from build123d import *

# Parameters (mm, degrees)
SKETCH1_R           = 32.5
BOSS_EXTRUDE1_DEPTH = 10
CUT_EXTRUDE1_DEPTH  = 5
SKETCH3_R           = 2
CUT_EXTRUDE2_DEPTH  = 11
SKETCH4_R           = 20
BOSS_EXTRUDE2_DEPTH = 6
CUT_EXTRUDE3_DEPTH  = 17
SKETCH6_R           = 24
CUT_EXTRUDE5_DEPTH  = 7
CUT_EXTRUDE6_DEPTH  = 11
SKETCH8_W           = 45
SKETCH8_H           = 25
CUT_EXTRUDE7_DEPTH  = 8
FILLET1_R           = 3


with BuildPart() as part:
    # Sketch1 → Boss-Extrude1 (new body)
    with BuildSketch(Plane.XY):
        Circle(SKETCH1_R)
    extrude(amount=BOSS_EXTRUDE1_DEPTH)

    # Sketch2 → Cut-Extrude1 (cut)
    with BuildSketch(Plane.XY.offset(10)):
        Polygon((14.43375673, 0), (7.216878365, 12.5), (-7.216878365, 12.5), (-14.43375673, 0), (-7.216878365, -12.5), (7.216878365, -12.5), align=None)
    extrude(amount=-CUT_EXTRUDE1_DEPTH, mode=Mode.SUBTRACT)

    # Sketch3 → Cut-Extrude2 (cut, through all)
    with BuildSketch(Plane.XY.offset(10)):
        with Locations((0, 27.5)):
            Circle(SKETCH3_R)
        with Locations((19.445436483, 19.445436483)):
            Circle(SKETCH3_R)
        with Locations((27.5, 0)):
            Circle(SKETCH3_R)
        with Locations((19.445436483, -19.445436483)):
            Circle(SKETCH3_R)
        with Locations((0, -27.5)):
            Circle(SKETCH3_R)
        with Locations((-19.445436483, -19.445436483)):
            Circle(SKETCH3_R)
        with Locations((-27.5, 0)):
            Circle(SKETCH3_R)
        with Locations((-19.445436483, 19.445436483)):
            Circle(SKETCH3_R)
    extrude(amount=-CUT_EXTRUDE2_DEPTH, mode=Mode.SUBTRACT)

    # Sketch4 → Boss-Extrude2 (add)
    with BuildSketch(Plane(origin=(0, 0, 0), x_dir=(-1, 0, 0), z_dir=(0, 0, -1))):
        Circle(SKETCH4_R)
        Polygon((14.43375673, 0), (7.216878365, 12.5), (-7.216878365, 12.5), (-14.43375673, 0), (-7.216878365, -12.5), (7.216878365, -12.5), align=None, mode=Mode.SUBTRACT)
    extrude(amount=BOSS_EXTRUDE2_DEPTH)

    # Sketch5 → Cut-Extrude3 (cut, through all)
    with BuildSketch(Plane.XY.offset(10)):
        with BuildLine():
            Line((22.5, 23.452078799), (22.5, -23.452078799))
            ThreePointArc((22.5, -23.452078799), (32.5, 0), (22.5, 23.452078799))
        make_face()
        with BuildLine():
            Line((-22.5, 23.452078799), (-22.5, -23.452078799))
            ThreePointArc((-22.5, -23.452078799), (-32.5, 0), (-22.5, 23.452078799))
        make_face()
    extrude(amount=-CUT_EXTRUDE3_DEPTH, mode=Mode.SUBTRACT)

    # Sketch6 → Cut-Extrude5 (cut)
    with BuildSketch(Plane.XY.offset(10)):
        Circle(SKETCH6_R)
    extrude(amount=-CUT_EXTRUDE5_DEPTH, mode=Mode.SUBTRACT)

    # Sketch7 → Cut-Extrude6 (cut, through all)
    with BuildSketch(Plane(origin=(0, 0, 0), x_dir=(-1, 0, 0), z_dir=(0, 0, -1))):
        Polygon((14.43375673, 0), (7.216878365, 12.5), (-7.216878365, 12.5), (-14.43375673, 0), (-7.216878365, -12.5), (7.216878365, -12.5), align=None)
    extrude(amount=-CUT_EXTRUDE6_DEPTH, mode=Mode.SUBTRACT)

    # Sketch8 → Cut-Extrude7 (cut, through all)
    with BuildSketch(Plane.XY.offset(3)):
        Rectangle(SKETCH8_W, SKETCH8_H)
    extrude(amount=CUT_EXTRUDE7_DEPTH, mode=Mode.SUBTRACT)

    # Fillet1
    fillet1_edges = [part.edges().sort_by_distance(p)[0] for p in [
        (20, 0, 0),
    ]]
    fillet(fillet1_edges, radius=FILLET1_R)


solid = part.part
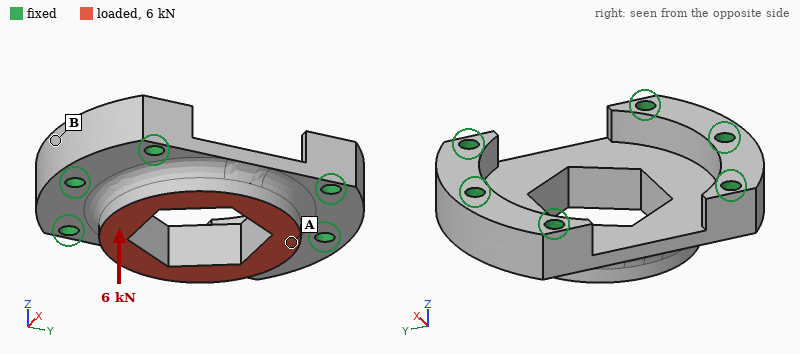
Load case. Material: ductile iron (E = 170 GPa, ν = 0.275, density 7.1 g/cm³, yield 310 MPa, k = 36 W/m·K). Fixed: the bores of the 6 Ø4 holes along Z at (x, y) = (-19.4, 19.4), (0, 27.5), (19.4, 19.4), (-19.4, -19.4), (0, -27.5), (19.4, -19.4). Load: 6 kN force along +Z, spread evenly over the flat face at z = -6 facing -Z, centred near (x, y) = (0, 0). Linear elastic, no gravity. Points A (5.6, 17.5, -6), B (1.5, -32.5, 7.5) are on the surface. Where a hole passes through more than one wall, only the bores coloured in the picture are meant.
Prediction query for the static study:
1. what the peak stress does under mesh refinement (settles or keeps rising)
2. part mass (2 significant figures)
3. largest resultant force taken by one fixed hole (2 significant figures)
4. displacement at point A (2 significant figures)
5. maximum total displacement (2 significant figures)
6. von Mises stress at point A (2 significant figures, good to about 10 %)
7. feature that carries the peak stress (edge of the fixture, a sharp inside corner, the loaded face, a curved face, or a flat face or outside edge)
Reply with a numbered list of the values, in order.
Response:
1. keeps rising
2. 120 g
3. 1.6 kN
4. 8.5 µm
5. 13 µm
6. 28 MPa
7. a sharp inside corner
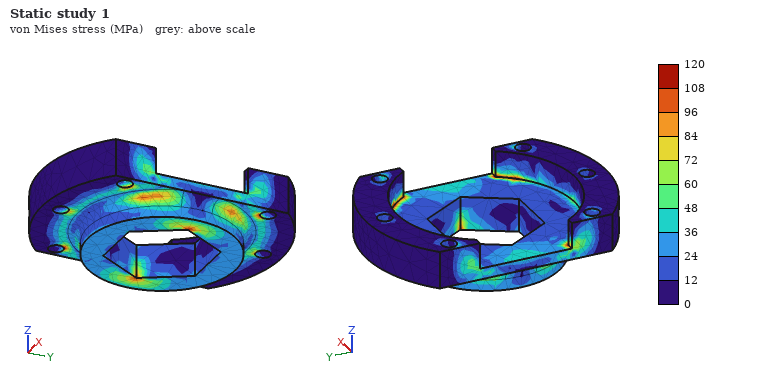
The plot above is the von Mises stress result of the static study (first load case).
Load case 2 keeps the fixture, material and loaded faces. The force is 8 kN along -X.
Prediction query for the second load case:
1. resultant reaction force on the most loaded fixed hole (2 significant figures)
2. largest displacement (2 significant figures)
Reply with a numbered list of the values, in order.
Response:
1. 1.8 kN
2. 12 µm
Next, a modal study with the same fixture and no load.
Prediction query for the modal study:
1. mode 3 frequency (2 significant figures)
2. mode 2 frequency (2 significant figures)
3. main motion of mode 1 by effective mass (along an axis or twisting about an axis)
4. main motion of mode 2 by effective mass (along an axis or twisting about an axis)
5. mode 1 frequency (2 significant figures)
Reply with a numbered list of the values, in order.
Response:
1. 26 kHz
2. 19 kHz
3. along Z
4. twisting about Y
5. 17 kHz
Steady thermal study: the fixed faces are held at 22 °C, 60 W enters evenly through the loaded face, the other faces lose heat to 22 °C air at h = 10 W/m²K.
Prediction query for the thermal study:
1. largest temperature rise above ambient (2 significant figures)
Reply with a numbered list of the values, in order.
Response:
1. 65 K
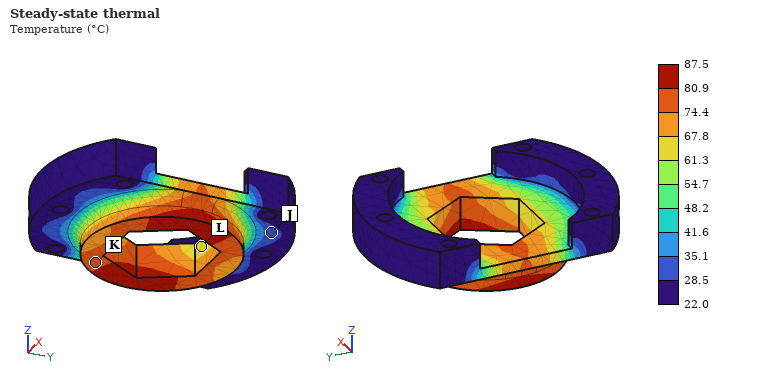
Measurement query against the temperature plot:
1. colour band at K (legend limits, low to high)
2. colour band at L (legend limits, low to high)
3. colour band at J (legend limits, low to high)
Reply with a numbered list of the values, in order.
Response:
1. 74.4 to 80.9 °C
2. 61.3 to 67.8 °C
3. 28.5 to 35.1 °C
